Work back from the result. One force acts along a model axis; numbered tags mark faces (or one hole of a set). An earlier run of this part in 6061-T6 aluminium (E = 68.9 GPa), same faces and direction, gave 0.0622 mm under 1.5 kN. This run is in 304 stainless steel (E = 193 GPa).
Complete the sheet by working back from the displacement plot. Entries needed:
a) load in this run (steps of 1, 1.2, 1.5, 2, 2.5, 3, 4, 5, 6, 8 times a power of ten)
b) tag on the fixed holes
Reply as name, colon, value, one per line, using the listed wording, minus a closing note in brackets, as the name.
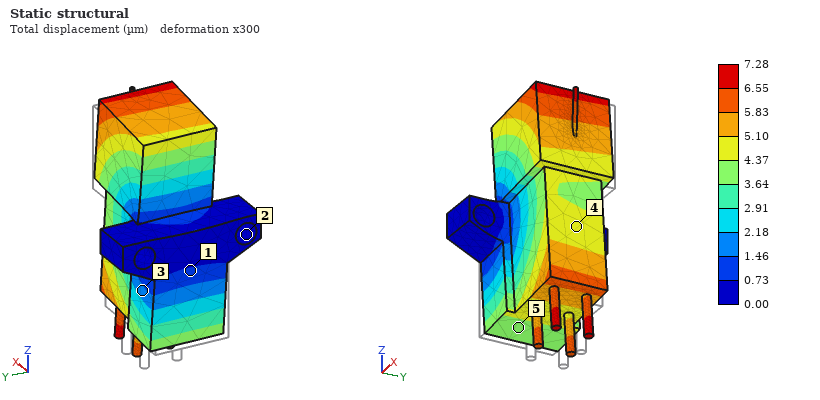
load in this run: 500 N
tag on the fixed holes: 2
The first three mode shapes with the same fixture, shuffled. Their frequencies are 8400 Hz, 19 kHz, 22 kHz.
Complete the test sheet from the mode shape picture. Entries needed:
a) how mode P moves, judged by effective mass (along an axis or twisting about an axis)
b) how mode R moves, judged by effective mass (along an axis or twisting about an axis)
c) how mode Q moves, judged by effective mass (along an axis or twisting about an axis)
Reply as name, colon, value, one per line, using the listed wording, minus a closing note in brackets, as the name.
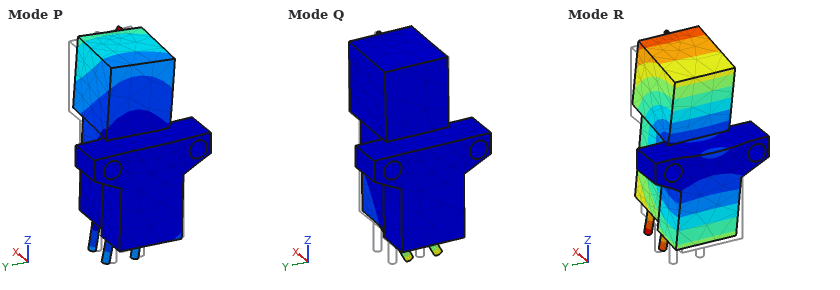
how mode P moves, judged by effective mass: along Y
how mode R moves, judged by effective mass: along Z
how mode Q moves, judged by effective mass: along Y
